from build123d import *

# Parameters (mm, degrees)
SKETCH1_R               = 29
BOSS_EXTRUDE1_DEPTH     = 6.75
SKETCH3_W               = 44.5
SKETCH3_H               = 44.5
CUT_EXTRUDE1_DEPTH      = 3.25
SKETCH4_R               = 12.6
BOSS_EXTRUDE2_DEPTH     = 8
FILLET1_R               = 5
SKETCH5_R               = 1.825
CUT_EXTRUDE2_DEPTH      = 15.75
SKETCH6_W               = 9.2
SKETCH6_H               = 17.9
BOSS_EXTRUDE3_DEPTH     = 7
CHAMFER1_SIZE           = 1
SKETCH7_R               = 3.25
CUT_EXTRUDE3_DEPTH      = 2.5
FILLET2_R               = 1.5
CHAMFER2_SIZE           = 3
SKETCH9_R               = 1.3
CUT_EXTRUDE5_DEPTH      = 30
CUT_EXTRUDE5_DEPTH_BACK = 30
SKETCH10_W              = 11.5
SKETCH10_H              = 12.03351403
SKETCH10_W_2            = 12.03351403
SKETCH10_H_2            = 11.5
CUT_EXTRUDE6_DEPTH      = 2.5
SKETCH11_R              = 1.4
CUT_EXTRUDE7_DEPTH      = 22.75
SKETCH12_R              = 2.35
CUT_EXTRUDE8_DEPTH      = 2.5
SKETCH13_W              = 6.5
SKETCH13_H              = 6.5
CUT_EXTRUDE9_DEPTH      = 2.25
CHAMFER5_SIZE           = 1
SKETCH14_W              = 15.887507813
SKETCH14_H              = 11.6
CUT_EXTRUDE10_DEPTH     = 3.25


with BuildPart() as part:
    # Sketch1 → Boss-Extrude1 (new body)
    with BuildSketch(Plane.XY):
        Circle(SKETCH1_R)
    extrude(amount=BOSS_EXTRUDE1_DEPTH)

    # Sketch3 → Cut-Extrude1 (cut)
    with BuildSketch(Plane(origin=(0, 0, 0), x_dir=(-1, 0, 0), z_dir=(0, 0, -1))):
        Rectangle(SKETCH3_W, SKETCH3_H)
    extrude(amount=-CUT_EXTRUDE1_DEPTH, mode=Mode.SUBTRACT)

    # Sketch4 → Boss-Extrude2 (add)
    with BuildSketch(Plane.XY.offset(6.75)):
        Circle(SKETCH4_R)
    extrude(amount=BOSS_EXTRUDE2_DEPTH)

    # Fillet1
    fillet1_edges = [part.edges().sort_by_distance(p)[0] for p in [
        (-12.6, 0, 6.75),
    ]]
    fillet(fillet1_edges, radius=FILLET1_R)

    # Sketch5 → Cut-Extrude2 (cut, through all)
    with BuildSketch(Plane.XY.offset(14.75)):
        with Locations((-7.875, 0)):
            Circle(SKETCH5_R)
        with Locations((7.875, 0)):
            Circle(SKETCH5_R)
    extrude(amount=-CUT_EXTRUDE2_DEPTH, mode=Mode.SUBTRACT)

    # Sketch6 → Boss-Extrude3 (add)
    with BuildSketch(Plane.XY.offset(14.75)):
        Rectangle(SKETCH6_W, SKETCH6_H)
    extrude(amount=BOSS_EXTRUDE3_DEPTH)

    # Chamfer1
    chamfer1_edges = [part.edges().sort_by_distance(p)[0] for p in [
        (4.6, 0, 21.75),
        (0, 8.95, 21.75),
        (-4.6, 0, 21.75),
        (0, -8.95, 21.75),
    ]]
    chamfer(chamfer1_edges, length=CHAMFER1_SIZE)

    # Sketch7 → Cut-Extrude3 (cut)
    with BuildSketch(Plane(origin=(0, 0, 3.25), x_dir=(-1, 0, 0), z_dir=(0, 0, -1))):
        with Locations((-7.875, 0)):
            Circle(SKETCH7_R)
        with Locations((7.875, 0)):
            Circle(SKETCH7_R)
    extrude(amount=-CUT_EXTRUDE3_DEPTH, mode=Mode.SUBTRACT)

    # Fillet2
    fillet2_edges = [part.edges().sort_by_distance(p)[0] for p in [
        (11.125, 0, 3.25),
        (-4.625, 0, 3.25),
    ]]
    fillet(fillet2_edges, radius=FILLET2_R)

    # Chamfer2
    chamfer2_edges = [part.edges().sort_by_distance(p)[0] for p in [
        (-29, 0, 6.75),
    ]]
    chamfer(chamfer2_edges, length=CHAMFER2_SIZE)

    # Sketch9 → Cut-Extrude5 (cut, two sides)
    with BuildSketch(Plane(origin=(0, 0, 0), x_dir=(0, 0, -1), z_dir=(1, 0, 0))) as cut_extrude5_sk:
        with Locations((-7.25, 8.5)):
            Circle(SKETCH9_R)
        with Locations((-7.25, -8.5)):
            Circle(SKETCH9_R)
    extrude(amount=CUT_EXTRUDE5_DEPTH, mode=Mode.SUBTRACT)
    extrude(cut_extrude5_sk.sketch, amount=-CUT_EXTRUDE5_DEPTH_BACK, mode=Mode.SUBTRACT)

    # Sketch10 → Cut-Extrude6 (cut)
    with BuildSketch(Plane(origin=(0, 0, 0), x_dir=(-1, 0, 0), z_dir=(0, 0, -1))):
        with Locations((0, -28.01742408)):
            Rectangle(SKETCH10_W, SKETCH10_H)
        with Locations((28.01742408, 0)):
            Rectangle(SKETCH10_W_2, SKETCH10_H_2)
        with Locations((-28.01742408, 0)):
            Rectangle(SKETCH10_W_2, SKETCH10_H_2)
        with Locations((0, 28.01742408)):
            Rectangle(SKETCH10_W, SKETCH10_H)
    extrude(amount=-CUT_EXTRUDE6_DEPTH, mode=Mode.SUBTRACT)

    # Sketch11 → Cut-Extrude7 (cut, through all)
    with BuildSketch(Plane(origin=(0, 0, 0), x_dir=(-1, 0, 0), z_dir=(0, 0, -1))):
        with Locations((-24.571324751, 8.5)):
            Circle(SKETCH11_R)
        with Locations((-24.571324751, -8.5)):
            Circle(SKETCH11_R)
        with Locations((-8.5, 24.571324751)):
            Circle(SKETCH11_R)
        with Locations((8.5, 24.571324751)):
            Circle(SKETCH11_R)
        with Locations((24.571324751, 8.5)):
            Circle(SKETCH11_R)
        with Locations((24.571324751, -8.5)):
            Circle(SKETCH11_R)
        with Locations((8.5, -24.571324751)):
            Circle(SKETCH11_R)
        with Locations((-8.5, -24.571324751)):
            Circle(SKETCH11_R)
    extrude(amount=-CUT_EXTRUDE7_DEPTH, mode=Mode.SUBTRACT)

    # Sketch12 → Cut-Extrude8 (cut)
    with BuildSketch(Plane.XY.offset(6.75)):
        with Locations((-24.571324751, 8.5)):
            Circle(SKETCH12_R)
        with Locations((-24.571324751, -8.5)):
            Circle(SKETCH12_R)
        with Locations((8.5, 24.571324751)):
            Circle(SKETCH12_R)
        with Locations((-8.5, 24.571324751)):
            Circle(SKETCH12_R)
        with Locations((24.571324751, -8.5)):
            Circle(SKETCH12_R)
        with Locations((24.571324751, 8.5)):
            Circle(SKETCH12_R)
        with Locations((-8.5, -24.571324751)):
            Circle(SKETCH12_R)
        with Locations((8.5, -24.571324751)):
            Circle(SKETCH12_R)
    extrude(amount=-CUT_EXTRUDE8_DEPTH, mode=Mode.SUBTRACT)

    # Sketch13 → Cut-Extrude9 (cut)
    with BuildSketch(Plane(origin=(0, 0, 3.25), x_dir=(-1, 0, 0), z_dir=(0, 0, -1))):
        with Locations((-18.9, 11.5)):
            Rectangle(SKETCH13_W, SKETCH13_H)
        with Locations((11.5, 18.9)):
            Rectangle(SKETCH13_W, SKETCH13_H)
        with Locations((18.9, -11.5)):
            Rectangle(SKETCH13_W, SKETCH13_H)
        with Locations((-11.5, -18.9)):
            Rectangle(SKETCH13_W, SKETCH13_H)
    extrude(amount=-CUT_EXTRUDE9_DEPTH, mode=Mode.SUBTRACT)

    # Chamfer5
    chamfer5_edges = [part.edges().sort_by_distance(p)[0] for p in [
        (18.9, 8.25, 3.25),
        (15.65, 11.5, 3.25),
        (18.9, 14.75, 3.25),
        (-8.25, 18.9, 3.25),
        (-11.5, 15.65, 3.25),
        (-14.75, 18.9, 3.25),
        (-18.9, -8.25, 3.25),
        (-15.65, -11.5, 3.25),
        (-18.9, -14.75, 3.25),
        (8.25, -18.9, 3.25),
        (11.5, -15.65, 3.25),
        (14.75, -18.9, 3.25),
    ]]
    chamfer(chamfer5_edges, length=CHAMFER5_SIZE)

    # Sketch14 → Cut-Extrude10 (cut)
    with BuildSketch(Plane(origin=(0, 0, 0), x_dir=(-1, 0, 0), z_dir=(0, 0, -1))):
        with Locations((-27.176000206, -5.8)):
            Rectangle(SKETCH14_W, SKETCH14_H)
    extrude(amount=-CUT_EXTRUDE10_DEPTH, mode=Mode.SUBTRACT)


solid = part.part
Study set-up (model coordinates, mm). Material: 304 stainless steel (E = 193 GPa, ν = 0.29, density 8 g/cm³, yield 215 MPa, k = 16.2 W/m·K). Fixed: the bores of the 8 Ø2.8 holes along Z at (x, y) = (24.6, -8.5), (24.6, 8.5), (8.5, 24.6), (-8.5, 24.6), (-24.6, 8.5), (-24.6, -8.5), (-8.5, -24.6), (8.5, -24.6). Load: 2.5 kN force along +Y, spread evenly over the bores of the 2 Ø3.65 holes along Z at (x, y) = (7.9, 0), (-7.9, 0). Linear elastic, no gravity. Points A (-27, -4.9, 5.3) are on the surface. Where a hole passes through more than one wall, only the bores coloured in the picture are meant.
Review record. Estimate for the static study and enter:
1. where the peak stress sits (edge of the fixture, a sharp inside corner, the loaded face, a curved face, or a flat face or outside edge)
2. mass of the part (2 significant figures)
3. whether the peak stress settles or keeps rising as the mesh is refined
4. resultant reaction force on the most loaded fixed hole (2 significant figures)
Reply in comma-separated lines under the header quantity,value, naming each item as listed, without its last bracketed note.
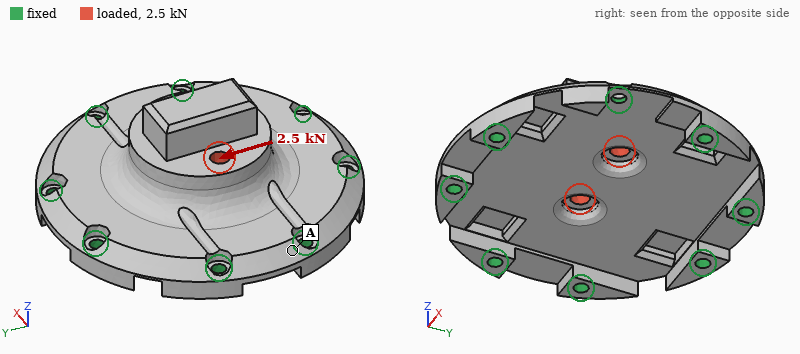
quantity,value
where the peak stress sits,a sharp inside corner
mass of the part,110 g
whether the peak stress settles or keeps rising as the mesh is refined,keeps rising
resultant reaction force on the most loaded fixed hole,560 N
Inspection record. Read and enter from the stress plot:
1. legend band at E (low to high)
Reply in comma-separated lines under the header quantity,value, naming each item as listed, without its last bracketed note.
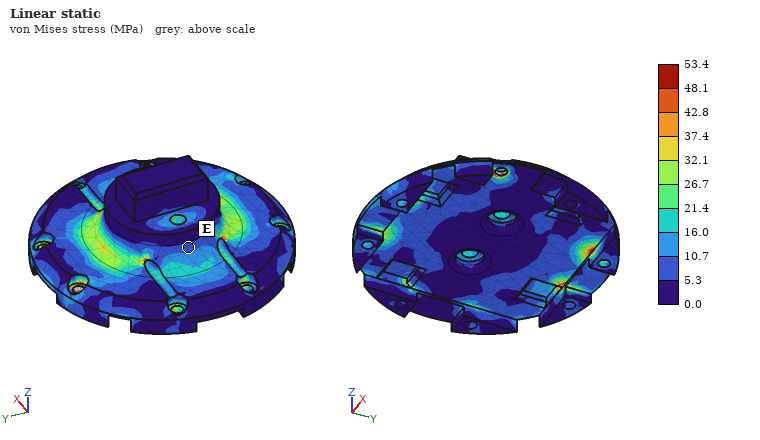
quantity,value
legend band at E,5.3 to 10.7 MPa
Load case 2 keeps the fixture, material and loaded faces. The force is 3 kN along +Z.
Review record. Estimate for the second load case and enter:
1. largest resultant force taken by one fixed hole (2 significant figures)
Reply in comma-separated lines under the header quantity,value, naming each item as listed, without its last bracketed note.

quantity,value
largest resultant force taken by one fixed hole,850 N
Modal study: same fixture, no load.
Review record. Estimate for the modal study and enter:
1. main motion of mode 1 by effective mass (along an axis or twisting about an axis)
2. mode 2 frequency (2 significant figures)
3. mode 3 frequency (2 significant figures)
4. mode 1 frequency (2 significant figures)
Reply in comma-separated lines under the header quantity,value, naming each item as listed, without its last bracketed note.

quantity,value
main motion of mode 1 by effective mass,along Z
mode 2 frequency,15 kHz
mode 3 frequency,16 kHz
mode 1 frequency,9900 Hz
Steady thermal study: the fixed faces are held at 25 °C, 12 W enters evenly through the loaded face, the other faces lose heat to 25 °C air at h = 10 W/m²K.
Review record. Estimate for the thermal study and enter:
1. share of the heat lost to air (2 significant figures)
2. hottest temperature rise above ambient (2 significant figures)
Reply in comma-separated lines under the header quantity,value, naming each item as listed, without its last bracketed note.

quantity,value
share of the heat lost to air,13 %
hottest temperature rise above ambient,49 K
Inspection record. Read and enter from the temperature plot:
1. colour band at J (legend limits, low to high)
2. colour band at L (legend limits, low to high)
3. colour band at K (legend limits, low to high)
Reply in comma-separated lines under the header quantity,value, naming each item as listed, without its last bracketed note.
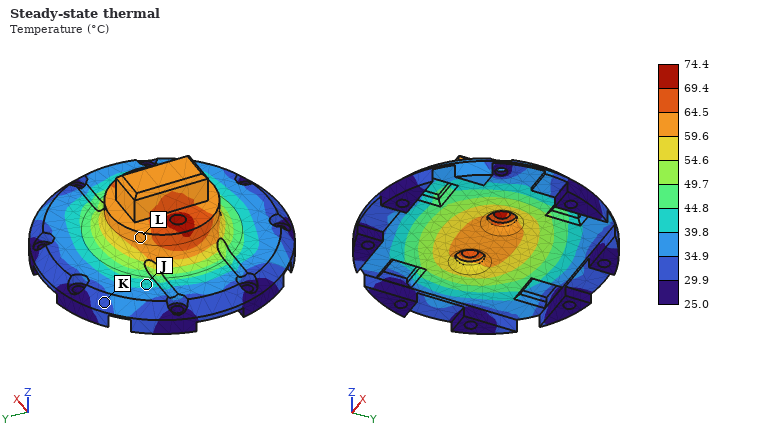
quantity,value
colour band at J,39.8 to 44.8 °C
colour band at L,59.6 to 64.5 °C
colour band at K,29.9 to 34.9 °C
